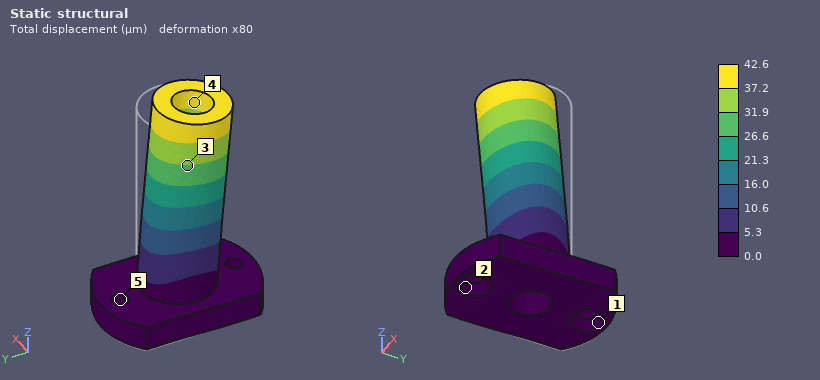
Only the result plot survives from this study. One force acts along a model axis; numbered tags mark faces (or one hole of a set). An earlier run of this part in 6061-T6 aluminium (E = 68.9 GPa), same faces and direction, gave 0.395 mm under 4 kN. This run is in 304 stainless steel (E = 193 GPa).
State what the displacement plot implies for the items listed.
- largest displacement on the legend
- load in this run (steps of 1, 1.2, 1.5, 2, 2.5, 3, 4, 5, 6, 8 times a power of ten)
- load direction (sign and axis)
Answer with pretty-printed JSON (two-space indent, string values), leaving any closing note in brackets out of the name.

{
  "largest displacement on the legend": "42.6 µm",
  "load in this run": "1.2 kN",
  "load direction": "-Y"
}
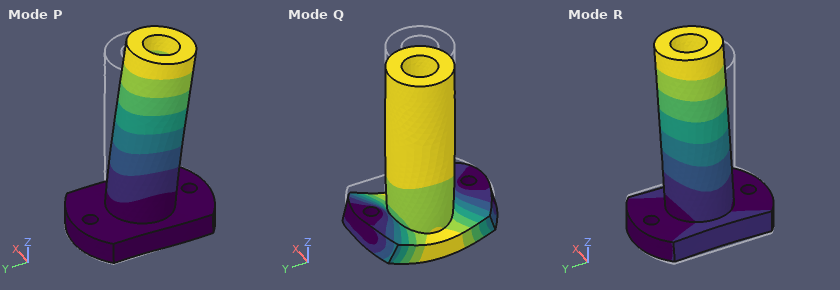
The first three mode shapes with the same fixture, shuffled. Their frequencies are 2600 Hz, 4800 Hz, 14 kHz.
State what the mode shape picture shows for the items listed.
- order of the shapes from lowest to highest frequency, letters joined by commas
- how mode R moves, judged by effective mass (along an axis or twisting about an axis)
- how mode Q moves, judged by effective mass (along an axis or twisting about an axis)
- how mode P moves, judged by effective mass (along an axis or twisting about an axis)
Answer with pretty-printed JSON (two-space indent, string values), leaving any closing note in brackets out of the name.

{
  "order of the shapes from lowest to highest frequency, letters joined by commas": "R, P, Q",
  "how mode R moves, judged by effective mass": "along X",
  "how mode Q moves, judged by effective mass": "along Z",
  "how mode P moves, judged by effective mass": "along Y"
}
